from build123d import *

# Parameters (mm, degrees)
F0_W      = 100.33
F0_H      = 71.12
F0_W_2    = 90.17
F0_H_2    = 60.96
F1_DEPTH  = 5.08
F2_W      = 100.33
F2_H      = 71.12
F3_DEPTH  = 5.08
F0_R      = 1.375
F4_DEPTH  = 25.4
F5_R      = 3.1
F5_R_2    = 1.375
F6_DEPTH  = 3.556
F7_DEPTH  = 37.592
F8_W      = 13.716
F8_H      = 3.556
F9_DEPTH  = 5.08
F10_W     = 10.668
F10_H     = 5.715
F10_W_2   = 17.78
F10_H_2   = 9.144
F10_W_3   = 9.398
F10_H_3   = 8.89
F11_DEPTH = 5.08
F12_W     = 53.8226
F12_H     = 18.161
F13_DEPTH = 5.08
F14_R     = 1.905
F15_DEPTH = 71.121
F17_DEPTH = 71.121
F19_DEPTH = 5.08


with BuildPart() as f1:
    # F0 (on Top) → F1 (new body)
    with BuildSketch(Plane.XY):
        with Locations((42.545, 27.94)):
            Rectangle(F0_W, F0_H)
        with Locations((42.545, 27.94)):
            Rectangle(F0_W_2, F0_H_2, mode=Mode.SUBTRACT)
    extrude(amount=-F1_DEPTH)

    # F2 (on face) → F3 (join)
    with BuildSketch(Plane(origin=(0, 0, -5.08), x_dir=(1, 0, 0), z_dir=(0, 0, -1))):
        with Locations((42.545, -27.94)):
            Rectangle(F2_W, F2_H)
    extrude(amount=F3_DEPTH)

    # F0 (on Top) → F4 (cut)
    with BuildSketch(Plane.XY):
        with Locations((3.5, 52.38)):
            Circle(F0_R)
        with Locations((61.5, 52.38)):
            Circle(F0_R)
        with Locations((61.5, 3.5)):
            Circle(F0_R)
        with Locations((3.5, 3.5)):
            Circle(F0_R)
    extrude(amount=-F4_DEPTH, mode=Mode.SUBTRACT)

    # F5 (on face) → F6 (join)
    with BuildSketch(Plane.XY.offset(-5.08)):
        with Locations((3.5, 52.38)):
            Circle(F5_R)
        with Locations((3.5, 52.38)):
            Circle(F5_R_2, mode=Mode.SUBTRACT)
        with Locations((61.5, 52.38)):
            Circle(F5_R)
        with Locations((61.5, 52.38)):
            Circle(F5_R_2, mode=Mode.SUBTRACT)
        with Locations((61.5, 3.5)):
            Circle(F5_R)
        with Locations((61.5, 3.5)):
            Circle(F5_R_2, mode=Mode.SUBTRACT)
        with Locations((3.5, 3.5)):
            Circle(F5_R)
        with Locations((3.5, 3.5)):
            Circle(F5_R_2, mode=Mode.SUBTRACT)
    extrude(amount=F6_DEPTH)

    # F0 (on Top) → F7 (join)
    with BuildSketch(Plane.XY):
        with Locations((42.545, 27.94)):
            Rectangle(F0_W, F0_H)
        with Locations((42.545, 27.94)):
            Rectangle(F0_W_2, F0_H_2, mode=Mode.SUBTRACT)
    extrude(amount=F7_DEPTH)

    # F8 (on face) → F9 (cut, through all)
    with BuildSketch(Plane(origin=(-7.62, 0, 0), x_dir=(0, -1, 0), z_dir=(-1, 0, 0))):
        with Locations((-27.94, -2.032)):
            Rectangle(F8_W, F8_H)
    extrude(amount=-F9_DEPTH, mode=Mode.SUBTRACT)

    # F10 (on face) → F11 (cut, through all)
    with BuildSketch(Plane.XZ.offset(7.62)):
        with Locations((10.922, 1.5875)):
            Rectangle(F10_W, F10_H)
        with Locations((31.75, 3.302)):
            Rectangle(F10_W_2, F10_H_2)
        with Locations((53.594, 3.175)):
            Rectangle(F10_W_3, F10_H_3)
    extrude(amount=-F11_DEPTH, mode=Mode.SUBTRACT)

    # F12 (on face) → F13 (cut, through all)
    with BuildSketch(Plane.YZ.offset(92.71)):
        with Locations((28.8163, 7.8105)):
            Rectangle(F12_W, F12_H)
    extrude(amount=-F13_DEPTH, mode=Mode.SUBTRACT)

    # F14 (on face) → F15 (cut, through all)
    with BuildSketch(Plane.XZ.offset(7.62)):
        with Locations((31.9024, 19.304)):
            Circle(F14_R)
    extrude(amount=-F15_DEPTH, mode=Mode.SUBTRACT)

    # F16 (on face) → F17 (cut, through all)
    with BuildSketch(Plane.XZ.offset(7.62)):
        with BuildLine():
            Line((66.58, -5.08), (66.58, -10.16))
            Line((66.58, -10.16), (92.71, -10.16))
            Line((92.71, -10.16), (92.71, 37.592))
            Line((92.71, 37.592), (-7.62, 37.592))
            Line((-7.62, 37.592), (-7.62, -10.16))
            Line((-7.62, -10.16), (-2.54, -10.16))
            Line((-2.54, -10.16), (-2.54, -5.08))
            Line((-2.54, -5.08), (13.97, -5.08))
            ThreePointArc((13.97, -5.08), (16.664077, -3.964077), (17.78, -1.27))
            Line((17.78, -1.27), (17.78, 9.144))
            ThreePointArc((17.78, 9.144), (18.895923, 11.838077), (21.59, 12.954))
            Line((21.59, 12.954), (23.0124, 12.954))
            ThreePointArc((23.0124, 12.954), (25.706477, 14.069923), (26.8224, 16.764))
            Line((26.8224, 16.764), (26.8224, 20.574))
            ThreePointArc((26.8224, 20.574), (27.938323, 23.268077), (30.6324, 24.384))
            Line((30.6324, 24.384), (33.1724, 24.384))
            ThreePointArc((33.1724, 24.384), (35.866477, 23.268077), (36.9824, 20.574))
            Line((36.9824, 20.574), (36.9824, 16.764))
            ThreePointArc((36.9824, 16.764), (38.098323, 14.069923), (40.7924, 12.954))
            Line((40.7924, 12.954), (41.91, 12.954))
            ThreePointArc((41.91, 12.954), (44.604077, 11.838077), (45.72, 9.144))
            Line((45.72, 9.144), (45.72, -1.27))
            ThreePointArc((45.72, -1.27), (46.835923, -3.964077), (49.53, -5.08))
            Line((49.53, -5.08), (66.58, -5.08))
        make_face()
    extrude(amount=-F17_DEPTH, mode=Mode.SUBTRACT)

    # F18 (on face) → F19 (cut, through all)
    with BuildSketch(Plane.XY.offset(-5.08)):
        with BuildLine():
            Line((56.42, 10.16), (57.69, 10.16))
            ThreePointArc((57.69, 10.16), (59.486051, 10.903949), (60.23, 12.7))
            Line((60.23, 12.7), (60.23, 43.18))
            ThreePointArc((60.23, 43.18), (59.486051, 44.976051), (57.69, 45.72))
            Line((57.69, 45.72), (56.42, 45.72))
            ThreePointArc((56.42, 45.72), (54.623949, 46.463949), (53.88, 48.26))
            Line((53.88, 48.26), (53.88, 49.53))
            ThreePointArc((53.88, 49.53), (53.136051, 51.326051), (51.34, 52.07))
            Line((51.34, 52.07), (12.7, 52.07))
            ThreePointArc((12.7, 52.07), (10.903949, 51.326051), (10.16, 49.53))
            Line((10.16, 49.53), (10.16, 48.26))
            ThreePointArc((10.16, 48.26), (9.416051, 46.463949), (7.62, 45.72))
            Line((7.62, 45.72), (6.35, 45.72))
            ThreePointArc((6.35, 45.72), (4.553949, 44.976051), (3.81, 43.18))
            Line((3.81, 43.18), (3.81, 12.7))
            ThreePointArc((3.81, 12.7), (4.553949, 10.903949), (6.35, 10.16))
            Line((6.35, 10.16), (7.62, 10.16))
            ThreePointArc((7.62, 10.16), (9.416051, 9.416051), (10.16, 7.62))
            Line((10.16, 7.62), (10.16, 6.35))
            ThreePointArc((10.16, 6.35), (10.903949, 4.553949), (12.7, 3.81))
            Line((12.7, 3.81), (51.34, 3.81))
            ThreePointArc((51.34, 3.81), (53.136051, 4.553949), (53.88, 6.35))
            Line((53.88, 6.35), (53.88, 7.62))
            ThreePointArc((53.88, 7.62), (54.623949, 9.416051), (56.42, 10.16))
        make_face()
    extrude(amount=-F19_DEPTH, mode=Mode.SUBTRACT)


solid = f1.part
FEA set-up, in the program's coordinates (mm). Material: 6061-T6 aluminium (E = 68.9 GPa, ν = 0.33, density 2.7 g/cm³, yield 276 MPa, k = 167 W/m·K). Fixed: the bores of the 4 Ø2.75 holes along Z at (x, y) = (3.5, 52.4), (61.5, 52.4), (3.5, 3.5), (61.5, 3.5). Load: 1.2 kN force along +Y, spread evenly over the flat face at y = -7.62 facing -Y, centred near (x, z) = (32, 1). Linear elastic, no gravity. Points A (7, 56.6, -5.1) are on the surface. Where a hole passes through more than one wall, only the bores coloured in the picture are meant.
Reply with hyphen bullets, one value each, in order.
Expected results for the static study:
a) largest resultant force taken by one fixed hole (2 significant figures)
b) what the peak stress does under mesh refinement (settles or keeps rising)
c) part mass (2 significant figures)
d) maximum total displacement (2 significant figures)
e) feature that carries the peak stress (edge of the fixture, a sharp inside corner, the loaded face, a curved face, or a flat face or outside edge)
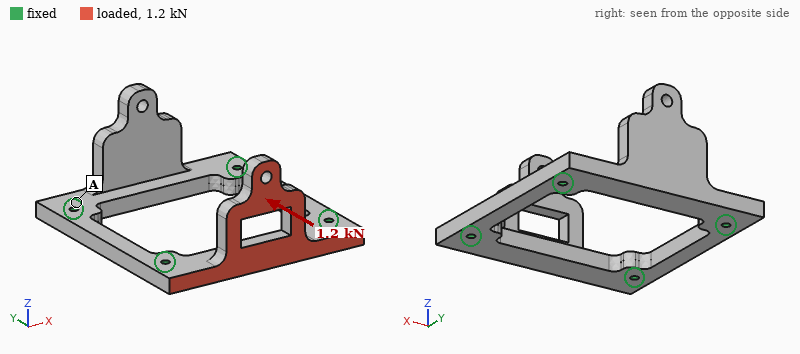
- 890 N
- keeps rising
- 47 g
- 0.55 mm
- edge of the fixture
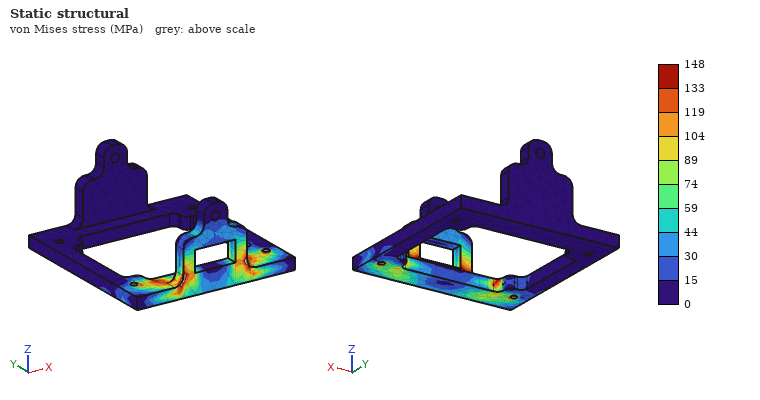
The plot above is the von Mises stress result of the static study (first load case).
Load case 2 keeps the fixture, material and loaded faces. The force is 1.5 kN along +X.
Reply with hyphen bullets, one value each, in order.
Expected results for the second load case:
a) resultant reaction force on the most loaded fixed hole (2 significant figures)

- 830 N
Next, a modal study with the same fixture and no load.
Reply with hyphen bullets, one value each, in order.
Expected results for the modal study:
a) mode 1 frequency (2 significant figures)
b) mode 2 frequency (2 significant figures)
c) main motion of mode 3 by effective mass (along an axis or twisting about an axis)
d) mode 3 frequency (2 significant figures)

- 2900 Hz
- 3000 Hz
- along Z
- 6400 Hz
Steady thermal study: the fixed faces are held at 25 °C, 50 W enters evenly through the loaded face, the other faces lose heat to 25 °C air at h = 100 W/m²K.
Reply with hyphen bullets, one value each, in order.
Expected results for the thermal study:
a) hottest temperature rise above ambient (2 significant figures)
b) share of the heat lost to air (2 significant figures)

- 64 K
- 20 %
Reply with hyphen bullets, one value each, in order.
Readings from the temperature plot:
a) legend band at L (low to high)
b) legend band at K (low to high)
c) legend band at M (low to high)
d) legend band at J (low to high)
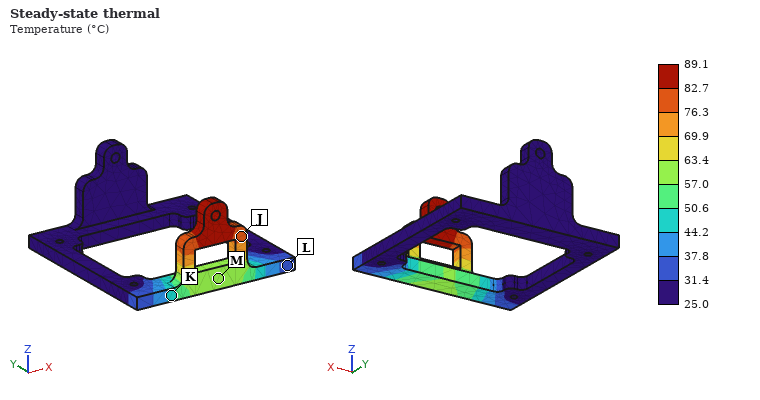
- 31.4 to 37.8 °C
- 44.2 to 50.6 °C
- 57.0 to 63.4 °C
- 76.3 to 82.7 °C
